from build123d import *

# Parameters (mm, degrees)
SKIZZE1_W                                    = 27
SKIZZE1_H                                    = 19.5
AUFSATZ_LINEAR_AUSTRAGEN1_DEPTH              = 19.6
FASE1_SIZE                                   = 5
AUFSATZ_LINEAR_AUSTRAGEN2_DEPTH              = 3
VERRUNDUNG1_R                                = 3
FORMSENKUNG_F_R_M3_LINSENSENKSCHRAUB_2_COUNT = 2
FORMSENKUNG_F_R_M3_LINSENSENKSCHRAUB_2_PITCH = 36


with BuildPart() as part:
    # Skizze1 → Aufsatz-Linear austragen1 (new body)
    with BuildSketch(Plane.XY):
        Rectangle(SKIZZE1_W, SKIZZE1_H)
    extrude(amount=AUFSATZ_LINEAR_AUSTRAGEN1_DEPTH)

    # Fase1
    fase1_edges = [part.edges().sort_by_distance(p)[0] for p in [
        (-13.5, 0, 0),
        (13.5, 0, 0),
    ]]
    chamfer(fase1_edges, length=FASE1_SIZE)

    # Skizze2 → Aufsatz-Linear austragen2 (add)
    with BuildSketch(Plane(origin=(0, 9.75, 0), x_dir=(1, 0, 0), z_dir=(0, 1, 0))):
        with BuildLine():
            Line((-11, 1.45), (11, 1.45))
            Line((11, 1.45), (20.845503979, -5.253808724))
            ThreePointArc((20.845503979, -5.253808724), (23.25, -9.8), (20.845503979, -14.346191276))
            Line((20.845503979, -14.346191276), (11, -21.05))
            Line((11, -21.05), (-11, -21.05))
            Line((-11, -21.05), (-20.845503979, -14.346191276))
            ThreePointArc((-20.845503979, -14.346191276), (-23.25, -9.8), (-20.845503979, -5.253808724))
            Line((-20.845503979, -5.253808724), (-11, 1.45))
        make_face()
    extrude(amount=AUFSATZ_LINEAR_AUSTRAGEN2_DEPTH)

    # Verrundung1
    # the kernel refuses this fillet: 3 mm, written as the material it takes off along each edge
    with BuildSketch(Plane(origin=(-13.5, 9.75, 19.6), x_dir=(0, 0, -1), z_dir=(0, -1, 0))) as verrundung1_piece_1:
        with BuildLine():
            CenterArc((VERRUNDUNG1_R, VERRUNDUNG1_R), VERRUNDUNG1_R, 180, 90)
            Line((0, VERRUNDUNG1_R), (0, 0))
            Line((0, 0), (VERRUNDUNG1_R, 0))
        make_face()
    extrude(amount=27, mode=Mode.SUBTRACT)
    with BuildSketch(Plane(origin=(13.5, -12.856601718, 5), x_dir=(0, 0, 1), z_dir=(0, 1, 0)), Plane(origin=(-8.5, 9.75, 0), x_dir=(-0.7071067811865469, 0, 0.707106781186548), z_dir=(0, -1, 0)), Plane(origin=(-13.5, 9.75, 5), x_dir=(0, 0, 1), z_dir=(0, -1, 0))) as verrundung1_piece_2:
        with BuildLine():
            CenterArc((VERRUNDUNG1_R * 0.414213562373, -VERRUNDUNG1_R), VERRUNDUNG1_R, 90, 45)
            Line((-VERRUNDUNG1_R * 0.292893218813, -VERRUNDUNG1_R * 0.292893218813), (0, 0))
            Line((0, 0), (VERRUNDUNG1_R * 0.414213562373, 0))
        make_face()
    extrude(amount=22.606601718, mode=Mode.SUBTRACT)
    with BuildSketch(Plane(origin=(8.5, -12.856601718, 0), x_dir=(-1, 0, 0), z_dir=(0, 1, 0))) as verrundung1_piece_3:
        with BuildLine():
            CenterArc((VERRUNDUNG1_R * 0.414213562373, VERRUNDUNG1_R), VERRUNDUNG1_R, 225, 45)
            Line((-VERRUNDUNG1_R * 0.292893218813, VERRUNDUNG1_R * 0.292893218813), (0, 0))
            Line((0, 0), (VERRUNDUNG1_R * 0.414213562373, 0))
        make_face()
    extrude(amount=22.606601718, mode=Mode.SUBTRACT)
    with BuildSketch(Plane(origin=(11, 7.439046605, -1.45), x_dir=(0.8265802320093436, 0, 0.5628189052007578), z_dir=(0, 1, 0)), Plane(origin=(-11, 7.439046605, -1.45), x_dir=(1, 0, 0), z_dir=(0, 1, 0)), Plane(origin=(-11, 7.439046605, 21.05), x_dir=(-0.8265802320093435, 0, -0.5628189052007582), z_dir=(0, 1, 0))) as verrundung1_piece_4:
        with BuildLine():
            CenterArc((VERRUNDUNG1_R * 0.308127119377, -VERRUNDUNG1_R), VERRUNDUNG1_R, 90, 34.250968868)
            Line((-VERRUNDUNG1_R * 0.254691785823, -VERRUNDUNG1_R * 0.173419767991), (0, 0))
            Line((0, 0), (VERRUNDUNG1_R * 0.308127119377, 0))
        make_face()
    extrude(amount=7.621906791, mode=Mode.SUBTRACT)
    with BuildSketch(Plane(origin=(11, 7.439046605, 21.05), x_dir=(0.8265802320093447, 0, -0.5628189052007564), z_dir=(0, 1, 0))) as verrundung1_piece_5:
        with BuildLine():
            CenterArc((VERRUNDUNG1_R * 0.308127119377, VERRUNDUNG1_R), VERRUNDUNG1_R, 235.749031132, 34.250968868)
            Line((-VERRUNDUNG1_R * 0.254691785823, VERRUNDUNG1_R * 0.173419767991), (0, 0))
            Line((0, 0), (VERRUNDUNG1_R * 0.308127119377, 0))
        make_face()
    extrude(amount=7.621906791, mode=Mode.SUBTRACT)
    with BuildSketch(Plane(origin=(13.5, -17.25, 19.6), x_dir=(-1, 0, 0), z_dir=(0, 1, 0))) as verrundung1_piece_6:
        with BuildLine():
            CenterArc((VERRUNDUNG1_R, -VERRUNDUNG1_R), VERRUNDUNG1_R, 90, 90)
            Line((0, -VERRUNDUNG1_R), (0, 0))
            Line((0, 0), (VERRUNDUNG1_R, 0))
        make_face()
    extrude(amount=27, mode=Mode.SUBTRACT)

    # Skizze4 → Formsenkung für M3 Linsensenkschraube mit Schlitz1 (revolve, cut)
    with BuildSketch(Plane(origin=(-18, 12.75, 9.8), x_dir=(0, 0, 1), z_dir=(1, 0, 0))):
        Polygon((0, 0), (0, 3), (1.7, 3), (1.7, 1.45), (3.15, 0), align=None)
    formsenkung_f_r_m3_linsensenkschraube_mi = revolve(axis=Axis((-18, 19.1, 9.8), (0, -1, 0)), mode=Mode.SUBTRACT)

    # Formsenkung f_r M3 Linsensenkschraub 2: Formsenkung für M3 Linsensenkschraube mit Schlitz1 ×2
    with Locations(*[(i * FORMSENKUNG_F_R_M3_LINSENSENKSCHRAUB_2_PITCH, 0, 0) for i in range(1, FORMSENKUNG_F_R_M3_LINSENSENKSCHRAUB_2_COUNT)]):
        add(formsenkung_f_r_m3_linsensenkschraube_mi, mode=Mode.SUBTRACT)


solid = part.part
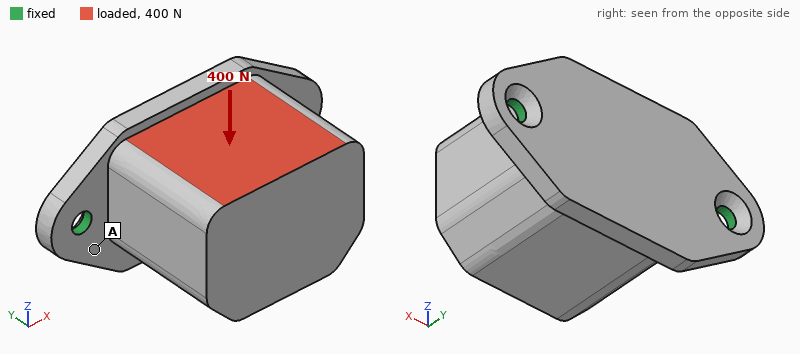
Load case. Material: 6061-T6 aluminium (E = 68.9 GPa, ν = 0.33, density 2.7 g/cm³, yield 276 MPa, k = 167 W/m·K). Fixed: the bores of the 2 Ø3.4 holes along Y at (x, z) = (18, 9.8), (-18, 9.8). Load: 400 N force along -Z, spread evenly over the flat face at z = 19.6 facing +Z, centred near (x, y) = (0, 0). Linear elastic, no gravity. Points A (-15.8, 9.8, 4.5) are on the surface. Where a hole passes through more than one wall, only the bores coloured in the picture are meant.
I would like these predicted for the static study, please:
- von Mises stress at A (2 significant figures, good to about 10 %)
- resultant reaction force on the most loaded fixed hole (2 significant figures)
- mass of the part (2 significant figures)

31 MPa
200 N
33 g
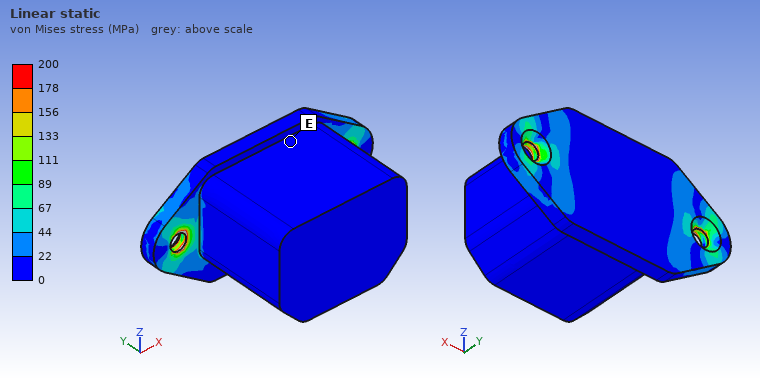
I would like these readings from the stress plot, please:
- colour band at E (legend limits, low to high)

0 to 22 MPa
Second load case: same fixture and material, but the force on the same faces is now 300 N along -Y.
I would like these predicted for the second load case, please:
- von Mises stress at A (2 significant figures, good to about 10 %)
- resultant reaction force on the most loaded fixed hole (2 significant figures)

18 MPa
150 N
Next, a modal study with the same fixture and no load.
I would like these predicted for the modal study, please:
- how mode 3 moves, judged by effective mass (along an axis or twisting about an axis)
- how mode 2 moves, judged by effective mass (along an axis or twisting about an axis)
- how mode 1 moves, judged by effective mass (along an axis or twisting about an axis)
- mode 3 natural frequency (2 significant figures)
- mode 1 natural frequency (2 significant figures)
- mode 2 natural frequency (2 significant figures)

along X
along Y
along Z
9000 Hz
2100 Hz
8200 Hz
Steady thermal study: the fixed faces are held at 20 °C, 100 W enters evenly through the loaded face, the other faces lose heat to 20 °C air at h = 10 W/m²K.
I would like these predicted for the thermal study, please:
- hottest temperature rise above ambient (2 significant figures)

78 K
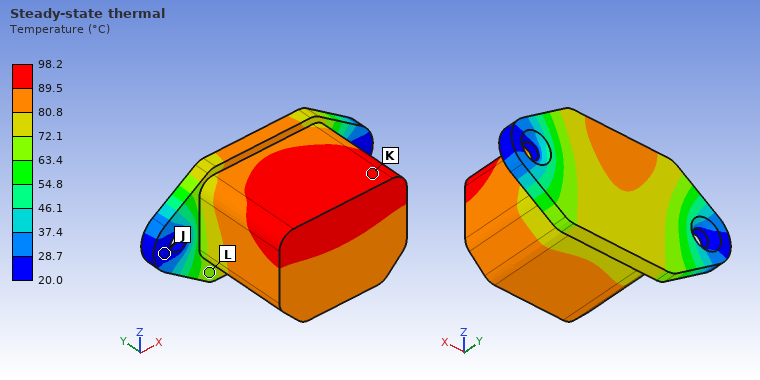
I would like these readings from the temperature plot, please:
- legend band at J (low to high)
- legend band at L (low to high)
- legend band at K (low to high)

20.0 to 28.7 °C
63.4 to 72.1 °C
89.5 to 98.2 °C
